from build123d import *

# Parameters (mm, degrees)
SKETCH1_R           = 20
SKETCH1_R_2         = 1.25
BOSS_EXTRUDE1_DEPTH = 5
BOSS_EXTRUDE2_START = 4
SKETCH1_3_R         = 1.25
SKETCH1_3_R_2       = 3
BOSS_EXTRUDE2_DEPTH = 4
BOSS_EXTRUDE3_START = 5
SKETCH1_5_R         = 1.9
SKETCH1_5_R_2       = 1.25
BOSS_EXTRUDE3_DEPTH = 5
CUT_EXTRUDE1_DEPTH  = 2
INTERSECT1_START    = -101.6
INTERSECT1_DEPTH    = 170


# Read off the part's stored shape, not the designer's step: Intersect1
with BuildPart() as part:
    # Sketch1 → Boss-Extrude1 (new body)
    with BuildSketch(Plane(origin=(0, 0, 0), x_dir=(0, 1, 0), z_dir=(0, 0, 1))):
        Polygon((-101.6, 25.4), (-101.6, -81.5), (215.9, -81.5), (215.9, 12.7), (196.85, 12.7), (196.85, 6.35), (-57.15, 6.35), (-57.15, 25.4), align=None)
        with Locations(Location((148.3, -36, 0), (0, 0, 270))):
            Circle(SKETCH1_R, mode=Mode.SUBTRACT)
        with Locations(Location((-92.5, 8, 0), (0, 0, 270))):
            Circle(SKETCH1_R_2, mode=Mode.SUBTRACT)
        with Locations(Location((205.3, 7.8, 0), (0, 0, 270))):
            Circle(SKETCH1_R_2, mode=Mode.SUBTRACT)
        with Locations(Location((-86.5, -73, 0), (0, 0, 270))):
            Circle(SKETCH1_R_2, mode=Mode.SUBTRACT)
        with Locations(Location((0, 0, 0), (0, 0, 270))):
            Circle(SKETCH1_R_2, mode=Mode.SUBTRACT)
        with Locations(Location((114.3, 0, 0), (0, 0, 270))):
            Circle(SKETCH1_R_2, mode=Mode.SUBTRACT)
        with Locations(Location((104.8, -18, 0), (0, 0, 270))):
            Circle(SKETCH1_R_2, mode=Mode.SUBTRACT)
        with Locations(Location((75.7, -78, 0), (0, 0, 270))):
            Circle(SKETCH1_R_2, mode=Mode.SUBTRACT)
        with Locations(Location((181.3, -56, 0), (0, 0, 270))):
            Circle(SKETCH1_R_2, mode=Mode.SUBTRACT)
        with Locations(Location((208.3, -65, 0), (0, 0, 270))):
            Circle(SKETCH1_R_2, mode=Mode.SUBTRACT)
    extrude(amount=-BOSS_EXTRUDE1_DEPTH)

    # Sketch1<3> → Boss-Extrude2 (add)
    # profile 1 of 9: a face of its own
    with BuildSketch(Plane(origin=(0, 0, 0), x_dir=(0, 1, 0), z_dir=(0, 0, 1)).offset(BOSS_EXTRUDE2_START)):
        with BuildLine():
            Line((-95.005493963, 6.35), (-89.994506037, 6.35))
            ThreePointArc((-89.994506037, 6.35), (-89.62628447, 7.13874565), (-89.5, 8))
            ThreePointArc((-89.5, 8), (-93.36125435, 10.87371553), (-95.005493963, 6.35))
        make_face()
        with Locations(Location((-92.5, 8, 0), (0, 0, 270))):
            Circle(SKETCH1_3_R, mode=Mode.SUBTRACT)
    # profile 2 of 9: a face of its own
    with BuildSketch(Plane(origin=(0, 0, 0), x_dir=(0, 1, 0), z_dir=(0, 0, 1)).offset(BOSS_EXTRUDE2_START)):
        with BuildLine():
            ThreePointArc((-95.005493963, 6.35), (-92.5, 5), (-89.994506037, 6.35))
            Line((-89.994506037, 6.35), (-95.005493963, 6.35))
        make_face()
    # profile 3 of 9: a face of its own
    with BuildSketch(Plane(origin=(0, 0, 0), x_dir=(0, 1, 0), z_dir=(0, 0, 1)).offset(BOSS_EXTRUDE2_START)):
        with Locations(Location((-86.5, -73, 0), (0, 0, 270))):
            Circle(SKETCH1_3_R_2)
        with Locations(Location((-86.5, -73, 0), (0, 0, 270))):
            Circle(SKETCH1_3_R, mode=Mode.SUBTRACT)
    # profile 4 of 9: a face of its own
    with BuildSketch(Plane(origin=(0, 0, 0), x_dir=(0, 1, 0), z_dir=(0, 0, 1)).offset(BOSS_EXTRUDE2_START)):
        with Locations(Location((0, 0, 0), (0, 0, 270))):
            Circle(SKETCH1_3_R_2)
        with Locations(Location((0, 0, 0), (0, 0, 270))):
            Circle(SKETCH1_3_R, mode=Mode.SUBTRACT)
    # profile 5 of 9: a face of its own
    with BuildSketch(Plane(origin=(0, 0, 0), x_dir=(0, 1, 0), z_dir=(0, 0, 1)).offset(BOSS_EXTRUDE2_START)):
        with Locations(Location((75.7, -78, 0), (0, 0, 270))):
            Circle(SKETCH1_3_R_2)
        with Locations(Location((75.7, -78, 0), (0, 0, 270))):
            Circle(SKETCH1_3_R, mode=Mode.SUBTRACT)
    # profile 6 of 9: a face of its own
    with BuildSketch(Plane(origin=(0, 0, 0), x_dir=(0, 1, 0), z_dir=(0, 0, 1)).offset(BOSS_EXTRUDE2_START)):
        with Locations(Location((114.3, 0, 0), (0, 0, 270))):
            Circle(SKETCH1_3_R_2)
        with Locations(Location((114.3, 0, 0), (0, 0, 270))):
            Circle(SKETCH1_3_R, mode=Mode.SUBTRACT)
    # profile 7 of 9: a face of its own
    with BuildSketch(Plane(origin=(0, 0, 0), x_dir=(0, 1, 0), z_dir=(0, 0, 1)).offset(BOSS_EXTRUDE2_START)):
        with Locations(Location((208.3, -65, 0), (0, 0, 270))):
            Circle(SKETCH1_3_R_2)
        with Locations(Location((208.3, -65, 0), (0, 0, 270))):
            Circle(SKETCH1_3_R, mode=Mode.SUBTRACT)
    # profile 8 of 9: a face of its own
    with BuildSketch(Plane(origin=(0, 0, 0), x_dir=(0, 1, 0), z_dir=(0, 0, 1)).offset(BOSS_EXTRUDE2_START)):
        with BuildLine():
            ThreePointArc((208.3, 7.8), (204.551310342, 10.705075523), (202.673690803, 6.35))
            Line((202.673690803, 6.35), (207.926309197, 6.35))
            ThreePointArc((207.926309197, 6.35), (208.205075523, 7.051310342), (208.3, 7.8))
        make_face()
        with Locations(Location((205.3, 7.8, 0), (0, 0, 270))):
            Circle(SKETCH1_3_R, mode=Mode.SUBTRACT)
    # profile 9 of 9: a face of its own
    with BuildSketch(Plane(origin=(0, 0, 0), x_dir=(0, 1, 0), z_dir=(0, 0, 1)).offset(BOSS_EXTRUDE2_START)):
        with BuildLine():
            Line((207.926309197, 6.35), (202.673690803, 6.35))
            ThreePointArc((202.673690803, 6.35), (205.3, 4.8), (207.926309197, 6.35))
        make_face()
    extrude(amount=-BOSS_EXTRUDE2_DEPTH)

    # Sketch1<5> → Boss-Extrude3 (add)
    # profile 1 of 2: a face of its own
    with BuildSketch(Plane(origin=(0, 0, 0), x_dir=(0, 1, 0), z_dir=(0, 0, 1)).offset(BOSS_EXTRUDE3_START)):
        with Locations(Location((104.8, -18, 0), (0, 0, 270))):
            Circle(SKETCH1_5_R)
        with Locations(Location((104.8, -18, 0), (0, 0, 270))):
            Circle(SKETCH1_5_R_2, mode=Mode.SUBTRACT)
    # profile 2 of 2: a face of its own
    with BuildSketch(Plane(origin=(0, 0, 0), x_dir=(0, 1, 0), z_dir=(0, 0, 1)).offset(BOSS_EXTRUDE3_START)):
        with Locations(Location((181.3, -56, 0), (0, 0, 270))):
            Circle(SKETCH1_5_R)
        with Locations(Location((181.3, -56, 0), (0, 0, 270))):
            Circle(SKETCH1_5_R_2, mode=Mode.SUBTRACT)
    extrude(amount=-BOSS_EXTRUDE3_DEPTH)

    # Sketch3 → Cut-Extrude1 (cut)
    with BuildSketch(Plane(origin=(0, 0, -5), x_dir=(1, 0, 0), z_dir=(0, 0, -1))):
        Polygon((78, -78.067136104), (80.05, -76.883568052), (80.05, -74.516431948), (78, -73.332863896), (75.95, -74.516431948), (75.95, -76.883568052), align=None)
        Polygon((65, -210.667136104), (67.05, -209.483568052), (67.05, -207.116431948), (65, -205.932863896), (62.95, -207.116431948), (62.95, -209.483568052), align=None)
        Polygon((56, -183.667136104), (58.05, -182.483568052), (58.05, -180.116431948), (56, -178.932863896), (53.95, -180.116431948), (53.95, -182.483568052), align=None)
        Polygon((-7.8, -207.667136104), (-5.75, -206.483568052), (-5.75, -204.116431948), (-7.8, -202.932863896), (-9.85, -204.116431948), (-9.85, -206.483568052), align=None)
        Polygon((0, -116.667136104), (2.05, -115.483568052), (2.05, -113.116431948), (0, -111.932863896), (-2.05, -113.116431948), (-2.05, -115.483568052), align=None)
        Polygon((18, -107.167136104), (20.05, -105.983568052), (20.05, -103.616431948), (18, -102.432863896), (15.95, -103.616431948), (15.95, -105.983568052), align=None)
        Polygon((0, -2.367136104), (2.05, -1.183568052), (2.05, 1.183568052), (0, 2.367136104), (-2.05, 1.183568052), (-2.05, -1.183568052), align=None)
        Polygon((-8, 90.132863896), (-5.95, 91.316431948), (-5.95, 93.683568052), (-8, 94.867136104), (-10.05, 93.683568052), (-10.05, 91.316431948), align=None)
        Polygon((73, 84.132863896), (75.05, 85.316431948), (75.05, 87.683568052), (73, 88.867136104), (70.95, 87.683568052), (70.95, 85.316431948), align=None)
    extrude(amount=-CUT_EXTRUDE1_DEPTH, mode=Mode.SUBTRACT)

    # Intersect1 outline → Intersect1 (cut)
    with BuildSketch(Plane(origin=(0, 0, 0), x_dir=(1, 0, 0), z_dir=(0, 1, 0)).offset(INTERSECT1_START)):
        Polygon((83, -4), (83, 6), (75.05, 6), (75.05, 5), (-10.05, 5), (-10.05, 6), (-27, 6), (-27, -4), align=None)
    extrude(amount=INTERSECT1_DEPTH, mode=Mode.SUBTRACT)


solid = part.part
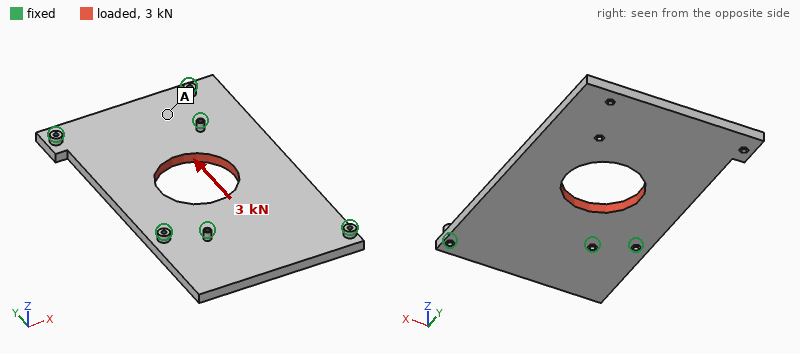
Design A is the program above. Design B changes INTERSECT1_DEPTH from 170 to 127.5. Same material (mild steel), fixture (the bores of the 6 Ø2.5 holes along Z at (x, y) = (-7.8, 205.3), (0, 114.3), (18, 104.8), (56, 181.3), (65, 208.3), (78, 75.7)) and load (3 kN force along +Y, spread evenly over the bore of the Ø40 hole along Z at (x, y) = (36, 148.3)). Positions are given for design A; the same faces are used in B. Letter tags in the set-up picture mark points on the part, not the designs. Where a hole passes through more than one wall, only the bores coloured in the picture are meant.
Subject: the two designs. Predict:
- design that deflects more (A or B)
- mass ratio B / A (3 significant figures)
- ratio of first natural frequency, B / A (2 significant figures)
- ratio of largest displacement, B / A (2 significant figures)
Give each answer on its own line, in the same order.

B
1.31
0.36
1.6
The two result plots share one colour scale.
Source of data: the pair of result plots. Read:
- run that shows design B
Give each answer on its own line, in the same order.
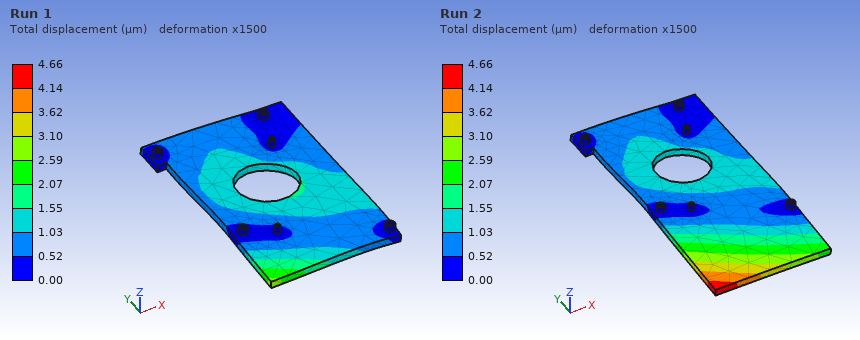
Run 2
